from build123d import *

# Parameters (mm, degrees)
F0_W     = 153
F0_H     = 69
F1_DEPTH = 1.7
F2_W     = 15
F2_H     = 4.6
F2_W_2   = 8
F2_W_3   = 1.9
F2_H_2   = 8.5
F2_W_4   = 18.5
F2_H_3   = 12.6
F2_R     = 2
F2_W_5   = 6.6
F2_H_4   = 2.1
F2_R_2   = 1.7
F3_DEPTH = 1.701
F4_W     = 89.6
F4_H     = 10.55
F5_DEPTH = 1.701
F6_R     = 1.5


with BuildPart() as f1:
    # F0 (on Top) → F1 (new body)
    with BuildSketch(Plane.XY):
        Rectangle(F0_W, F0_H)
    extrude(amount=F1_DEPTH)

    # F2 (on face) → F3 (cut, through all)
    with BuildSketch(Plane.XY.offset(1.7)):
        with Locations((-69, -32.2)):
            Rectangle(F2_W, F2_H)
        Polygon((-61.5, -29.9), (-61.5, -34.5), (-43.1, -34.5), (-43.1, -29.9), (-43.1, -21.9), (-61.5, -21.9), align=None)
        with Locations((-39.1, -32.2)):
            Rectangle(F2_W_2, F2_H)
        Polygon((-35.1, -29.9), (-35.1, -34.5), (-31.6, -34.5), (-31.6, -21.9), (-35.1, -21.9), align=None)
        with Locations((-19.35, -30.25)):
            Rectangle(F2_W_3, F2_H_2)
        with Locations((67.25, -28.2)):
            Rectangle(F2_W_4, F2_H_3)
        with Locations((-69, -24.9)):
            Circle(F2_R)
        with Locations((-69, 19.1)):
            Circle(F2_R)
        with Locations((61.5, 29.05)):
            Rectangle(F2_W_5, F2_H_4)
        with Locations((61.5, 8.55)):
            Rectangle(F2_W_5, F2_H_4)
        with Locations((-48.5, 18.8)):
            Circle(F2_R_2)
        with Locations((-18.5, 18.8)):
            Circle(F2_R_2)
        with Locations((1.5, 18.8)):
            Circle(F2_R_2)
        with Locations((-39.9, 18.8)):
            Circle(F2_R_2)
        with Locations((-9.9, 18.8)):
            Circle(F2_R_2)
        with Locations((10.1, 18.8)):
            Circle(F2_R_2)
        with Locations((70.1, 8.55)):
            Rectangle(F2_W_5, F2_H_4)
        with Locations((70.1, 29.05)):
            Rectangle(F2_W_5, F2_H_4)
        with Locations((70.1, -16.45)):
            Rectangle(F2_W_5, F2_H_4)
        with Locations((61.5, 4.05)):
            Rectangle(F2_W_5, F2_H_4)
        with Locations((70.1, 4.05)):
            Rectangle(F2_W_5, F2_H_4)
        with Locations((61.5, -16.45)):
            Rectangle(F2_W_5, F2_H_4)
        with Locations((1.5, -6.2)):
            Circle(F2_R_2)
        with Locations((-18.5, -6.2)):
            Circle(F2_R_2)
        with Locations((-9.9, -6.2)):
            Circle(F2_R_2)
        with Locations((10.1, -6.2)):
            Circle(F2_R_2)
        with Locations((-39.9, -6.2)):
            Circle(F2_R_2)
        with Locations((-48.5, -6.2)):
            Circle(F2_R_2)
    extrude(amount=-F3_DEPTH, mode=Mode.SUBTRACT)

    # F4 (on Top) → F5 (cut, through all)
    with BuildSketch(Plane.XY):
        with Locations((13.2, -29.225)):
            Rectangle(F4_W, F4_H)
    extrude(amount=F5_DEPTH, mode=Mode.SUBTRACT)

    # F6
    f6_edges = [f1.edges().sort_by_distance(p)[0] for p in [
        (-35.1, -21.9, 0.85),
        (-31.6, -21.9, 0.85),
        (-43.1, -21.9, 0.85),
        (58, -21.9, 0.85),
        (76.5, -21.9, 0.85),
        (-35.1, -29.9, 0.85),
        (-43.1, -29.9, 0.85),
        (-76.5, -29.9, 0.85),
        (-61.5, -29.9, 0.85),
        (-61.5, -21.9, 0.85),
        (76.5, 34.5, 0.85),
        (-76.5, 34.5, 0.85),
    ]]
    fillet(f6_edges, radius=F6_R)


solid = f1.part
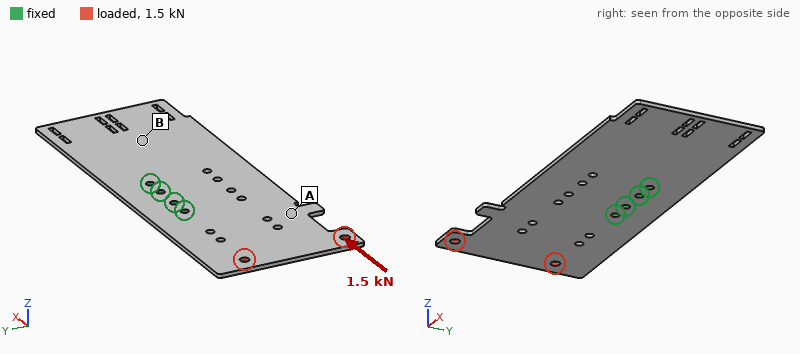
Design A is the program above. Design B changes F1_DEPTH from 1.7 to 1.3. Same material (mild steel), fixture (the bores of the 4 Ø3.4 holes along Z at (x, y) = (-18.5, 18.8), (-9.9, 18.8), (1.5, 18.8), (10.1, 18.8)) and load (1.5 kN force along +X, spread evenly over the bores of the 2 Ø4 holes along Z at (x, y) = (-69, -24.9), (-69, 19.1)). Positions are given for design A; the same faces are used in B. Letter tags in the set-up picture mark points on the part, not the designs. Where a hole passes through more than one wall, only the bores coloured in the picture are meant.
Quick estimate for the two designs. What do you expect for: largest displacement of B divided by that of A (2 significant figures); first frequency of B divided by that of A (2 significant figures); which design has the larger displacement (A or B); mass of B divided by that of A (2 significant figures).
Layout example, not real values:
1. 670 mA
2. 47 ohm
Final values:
1. 1.3
2. 0.77
3. B
4. 0.76
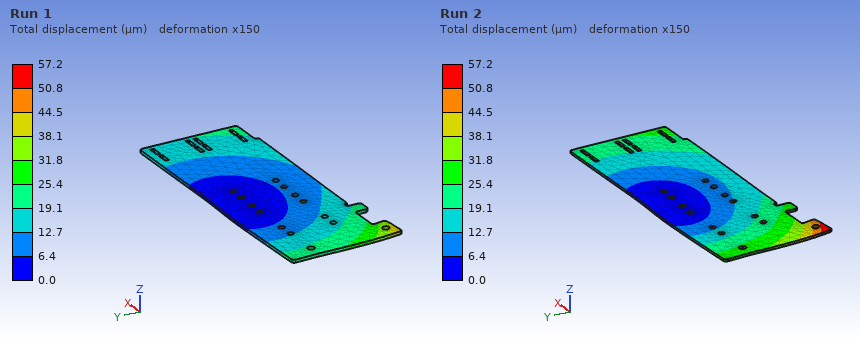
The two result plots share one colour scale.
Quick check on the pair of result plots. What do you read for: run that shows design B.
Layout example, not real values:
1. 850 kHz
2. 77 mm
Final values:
1. Run 2
